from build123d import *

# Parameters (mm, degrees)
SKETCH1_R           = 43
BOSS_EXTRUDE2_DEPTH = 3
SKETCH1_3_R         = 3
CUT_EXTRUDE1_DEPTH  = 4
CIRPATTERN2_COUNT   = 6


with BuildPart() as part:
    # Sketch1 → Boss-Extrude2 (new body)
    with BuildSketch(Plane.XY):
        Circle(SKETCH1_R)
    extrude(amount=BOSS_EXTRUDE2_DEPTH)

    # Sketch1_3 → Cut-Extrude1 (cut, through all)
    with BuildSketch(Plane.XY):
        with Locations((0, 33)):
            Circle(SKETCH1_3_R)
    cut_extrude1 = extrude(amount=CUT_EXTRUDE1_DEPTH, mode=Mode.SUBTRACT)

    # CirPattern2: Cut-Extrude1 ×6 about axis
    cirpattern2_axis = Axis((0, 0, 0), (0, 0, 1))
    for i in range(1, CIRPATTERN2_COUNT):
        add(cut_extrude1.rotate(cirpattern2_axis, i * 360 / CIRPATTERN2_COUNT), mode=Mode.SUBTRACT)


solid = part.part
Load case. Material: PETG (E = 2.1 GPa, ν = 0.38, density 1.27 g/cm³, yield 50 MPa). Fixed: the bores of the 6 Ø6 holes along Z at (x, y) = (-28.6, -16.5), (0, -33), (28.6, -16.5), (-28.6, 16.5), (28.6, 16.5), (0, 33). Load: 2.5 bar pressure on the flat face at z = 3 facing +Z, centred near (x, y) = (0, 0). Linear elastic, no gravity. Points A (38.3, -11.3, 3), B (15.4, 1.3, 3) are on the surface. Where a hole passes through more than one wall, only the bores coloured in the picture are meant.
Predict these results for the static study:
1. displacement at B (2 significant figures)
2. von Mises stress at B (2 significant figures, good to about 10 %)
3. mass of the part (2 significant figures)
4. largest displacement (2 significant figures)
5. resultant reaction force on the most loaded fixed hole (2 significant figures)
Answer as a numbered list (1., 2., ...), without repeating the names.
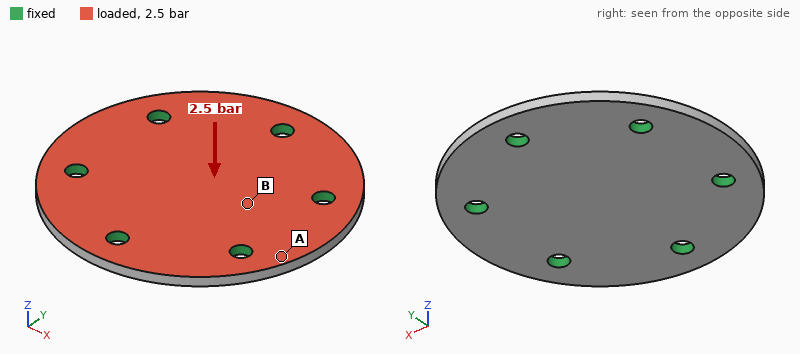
1. 0.52 mm
2. 8.9 MPa
3. 21 g
4. 0.82 mm
5. 240 N
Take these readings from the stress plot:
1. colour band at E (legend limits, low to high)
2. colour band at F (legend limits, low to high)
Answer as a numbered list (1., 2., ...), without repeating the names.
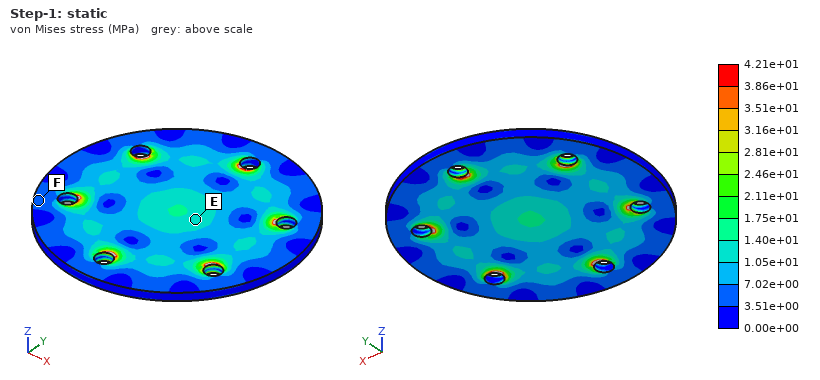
1. 1.05e+01 to 1.40e+01 MPa
2. 3.51e+00 to 7.02e+00 MPa
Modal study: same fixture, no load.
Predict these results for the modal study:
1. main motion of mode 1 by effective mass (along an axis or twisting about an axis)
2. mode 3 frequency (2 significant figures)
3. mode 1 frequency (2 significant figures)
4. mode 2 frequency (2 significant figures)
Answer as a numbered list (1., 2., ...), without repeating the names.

1. along Z
2. 3000 Hz
3. 1700 Hz
4. 2900 Hz
